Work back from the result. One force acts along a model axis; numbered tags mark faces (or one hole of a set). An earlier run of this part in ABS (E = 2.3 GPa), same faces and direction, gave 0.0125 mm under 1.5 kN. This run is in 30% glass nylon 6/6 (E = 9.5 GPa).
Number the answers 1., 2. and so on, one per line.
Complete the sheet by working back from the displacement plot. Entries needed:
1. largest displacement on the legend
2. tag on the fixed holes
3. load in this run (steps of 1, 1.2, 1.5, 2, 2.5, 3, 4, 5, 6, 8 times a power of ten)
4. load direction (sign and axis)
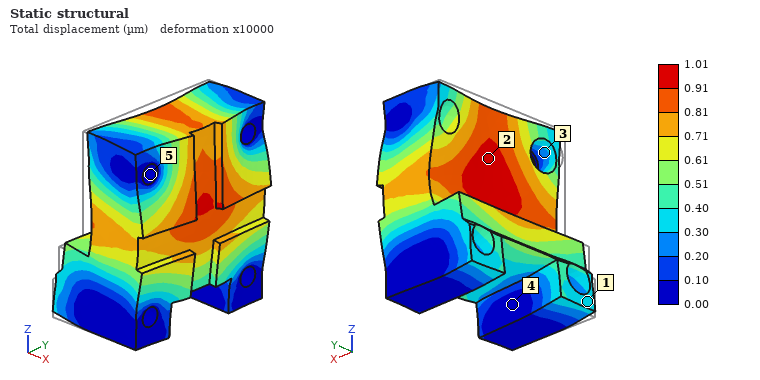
1. 1.01 µm
2. 5
3. 500 N
4. +X
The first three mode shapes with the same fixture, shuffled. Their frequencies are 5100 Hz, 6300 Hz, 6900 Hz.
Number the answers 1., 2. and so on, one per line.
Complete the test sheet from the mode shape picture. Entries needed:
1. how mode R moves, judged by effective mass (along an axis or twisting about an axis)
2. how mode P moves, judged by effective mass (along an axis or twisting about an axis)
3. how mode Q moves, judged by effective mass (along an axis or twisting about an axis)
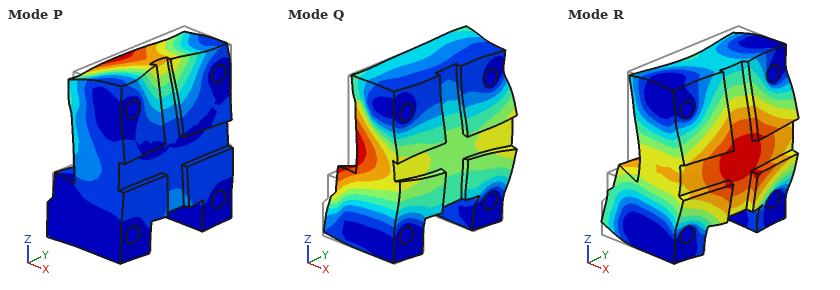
1. along X
2. along Z
3. along Y
